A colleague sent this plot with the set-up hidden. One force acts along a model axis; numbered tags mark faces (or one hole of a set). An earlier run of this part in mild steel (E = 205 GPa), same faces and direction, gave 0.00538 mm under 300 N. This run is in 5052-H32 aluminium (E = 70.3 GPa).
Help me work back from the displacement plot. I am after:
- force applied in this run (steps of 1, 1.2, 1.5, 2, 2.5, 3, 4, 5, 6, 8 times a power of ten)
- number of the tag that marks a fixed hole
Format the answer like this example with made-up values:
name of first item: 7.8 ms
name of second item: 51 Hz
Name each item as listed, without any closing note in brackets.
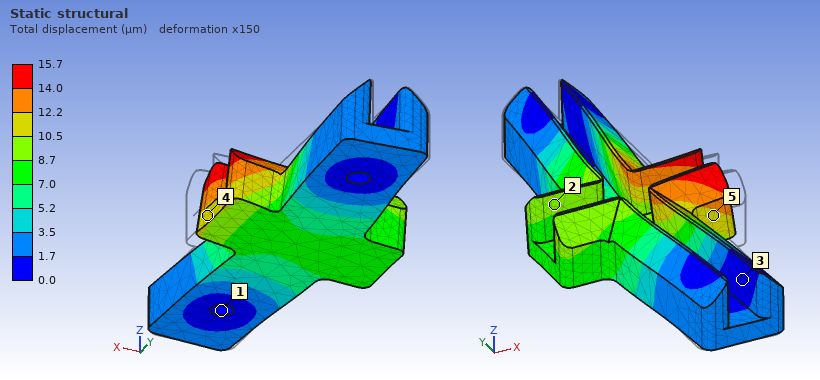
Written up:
force applied in this run: 300 N
number of the tag that marks a fixed hole: 1
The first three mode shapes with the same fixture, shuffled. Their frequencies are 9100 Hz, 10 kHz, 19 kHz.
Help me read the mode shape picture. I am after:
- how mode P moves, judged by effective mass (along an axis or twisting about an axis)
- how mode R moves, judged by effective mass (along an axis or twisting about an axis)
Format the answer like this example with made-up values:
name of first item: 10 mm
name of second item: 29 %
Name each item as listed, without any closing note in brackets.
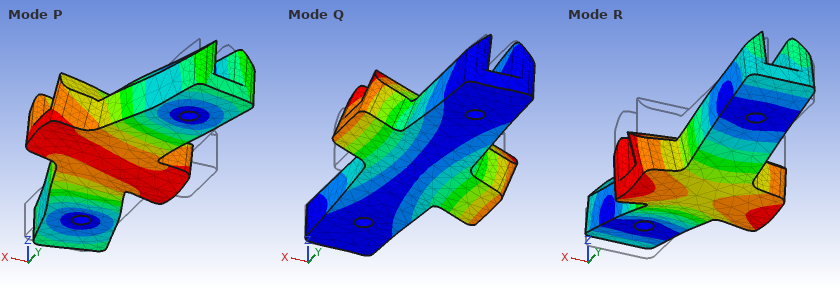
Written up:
how mode P moves, judged by effective mass: along X
how mode R moves, judged by effective mass: along Z
